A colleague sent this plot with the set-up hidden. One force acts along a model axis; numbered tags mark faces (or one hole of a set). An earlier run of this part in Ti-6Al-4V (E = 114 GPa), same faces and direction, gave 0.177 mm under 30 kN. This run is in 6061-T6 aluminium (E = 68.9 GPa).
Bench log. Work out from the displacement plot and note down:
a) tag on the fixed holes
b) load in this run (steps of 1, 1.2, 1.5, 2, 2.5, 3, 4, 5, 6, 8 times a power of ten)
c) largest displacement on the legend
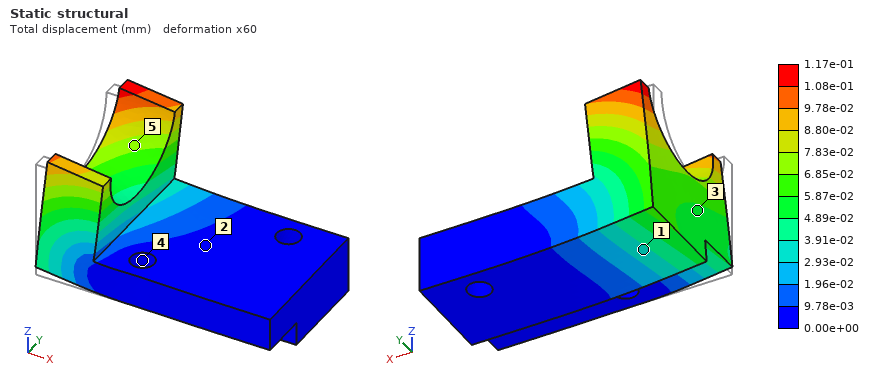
4
12 kN
1.17e-01 mm
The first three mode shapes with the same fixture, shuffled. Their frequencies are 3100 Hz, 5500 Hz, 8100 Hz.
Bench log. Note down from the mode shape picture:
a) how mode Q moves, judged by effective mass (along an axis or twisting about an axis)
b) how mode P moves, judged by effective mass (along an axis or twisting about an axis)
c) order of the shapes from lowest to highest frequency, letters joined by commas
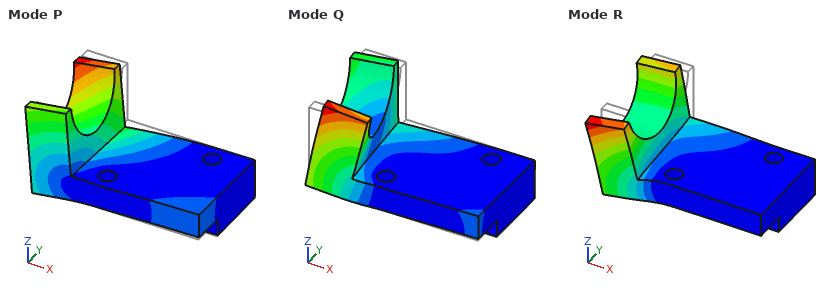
along Y
along Z
P, R, Q
